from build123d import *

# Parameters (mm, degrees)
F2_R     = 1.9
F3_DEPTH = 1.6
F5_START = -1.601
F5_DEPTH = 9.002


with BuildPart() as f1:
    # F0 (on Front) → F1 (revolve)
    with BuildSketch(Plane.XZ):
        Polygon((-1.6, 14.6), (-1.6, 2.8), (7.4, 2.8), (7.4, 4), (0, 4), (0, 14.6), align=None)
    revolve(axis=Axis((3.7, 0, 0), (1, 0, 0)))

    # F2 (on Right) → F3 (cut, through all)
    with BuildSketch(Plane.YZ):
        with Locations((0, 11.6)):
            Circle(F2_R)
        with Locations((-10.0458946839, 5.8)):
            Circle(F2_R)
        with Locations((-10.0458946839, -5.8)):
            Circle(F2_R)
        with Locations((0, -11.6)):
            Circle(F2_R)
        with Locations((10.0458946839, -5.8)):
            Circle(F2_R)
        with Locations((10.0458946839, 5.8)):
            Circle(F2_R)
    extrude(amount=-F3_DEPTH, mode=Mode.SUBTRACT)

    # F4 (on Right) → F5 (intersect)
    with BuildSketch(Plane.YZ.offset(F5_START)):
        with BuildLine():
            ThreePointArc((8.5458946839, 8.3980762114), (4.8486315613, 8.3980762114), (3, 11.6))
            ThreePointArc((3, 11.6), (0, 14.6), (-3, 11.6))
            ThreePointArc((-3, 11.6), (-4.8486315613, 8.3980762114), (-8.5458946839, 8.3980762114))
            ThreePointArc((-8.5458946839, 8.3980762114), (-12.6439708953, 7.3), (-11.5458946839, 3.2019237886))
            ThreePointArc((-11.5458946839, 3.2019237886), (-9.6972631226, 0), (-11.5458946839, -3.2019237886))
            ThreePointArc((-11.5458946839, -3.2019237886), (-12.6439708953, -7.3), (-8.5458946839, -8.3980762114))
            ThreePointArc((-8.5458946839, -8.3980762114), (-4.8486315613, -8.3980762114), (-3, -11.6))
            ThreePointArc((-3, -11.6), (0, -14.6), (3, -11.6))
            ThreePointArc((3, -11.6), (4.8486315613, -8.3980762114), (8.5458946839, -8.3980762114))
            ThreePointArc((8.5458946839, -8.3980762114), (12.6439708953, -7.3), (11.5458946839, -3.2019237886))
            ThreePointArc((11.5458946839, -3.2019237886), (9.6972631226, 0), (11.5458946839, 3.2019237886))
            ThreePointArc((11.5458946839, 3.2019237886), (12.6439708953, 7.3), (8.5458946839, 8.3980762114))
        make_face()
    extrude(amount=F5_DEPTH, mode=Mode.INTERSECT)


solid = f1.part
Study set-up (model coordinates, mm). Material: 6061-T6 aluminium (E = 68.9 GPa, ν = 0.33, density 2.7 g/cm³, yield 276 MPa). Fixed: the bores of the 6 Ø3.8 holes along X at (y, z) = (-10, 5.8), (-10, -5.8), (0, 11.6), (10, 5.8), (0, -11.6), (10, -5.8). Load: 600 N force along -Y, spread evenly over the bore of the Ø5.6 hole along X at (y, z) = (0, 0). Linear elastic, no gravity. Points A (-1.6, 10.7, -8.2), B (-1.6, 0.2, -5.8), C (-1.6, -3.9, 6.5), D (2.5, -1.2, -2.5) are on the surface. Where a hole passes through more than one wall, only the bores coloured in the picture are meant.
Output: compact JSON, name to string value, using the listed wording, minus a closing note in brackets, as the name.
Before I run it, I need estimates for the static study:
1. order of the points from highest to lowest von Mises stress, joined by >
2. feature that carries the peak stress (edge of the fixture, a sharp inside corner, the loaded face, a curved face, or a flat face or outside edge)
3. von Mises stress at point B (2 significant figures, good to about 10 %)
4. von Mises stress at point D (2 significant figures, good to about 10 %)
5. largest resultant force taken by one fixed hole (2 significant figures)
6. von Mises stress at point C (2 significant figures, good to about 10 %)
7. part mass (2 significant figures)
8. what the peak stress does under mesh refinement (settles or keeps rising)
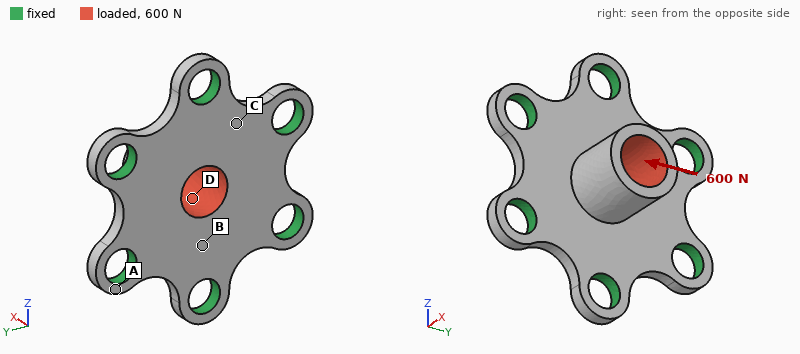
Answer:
{"order of the points from highest to lowest von Mises stress, joined by >": "D > B > C > A", "feature that carries the peak stress": "edge of the fixture", "von Mises stress at point B": "34 MPa", "von Mises stress at point D": "49 MPa", "largest resultant force taken by one fixed hole": "180 N", "von Mises stress at point C": "23 MPa", "part mass": "2.1 g", "what the peak stress does under mesh refinement": "keeps rising"}
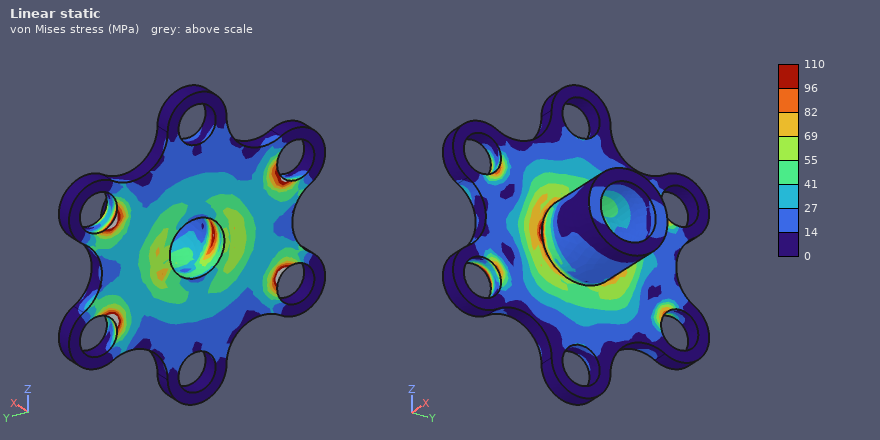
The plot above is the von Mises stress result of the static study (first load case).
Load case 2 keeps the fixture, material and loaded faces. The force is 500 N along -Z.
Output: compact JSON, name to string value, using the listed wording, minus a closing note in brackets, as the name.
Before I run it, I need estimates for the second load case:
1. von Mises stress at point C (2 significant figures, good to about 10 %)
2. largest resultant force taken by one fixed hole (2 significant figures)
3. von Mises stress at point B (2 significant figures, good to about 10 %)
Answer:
{"von Mises stress at point C": "22 MPa", "largest resultant force taken by one fixed hole": "170 N", "von Mises stress at point B": "32 MPa"}
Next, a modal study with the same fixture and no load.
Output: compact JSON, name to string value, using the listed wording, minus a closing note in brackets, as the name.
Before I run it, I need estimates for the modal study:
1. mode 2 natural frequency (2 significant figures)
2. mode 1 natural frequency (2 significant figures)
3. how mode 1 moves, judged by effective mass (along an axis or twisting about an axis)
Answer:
{"mode 2 natural frequency": "28 kHz", "mode 1 natural frequency": "26 kHz", "how mode 1 moves, judged by effective mass": "along X"}
